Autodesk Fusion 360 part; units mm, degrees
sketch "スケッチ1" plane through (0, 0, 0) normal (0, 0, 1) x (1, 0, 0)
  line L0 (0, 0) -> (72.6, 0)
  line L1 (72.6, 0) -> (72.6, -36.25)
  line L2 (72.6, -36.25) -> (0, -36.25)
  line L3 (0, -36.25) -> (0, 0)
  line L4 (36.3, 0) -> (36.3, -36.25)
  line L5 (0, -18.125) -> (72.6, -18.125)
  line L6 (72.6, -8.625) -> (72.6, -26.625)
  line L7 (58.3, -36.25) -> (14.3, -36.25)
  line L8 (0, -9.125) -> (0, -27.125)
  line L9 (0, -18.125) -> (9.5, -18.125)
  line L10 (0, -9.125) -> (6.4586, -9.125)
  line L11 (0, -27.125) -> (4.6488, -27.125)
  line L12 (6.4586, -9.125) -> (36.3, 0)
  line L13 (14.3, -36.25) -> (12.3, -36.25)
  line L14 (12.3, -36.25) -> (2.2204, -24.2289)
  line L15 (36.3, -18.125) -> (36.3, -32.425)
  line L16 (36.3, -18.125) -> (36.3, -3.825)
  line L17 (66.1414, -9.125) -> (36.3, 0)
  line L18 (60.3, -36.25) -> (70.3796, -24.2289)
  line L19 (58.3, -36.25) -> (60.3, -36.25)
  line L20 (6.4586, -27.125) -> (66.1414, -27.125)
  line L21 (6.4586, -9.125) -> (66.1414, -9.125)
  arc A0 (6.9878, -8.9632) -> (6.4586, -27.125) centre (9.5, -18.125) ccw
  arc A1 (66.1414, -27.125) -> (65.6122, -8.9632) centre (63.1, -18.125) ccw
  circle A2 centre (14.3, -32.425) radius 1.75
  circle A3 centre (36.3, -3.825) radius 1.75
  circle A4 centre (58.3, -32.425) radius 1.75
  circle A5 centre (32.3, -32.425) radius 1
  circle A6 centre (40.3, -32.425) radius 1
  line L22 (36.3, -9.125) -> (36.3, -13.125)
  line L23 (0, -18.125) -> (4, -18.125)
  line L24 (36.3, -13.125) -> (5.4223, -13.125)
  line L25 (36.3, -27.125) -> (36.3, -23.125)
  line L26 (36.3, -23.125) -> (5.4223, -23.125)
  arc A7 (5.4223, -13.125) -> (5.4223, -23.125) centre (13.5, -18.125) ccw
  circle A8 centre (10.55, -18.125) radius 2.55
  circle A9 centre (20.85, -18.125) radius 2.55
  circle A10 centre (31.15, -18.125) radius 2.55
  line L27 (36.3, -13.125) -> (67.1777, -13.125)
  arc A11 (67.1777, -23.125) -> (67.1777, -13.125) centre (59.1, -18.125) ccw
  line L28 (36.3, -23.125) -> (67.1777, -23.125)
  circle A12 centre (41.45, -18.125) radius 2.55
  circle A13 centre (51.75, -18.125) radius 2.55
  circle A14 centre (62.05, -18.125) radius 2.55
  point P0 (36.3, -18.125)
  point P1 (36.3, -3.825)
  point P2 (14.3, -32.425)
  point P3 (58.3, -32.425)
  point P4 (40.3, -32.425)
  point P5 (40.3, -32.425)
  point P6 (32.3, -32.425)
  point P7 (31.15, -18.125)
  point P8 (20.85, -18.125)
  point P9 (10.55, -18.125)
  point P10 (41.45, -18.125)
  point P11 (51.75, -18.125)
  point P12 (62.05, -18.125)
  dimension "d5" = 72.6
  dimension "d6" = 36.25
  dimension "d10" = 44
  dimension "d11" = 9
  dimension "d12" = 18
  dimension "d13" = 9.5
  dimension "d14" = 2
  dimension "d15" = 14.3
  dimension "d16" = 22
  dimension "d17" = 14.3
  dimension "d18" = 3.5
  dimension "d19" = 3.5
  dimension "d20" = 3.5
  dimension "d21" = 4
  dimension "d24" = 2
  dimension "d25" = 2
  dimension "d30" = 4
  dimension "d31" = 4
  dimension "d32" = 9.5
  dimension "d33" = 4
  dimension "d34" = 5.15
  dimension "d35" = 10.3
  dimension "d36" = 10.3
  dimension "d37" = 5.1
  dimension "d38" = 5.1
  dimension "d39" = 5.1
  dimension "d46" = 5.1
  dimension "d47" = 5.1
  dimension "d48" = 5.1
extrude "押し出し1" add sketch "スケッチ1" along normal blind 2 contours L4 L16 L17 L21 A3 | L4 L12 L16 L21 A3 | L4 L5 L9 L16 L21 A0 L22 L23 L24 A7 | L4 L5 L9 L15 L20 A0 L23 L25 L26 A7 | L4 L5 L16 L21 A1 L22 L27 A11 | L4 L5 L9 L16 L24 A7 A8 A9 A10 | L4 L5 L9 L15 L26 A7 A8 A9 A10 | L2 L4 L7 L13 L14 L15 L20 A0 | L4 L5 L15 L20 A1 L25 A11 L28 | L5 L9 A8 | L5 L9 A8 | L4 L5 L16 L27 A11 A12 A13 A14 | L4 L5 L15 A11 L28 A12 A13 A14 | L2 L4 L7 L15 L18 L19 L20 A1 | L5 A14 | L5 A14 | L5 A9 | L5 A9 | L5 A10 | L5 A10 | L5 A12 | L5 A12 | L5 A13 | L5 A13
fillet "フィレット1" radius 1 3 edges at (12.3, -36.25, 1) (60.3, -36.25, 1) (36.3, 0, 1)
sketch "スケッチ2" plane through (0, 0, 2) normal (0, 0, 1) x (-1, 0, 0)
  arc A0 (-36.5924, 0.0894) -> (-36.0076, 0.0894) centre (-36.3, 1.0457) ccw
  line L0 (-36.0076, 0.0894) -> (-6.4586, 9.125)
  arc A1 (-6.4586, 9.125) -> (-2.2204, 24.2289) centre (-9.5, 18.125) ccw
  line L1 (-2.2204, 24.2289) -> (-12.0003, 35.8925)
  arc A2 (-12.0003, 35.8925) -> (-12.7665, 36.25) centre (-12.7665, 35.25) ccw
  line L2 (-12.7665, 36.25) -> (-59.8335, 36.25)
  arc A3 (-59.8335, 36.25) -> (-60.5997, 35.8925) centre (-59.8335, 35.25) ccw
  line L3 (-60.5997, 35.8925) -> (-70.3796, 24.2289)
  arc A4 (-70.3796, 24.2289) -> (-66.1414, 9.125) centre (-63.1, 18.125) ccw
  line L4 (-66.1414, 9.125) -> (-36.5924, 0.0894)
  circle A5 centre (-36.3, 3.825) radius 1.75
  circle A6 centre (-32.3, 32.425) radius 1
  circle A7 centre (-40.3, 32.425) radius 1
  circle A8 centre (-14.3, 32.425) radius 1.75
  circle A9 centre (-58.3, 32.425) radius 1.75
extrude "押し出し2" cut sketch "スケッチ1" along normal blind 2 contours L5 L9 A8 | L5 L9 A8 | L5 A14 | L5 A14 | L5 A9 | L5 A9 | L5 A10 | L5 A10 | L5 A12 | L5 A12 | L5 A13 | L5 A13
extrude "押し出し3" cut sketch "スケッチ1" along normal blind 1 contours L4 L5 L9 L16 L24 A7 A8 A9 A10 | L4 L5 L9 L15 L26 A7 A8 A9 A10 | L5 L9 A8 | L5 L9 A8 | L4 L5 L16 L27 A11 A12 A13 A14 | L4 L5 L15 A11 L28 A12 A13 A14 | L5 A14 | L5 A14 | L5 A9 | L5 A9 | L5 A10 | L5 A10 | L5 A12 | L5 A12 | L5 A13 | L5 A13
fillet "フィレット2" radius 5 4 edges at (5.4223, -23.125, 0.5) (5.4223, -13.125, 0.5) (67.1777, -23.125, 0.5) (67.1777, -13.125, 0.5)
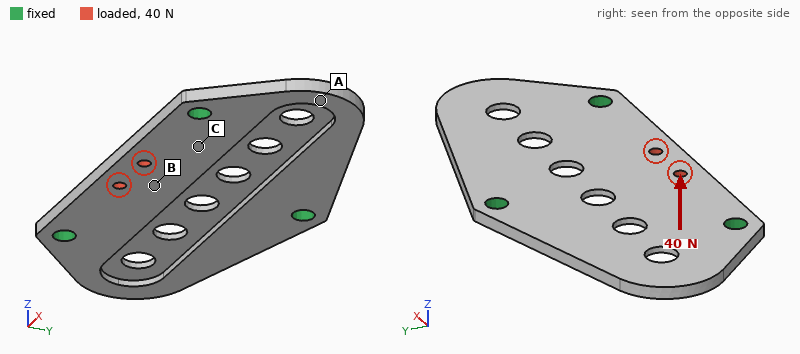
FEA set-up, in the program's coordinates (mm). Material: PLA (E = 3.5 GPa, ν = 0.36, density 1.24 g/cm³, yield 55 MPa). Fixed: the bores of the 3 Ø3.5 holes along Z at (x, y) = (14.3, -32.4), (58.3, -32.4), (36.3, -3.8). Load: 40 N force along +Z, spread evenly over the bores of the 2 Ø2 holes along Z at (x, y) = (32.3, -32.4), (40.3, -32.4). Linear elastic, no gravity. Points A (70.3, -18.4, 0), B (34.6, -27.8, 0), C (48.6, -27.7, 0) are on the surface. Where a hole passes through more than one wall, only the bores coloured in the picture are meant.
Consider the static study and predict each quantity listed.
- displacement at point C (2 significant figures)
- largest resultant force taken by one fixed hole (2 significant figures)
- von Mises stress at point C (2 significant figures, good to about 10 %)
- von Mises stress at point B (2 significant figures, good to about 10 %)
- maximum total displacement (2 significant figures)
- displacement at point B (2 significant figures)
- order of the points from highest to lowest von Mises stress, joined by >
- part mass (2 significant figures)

0.15 mm
19 N
7.7 MPa
12 MPa
0.58 mm
0.36 mm
B > C > A
4.0 g
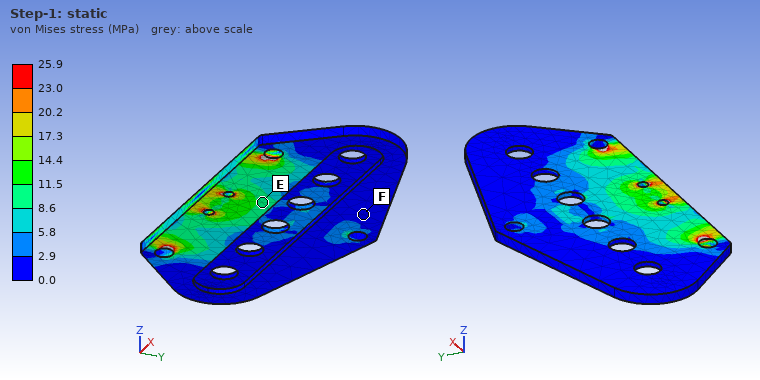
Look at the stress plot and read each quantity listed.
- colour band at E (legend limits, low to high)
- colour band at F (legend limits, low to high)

8.6 to 11.5 MPa
0.0 to 2.9 MPa
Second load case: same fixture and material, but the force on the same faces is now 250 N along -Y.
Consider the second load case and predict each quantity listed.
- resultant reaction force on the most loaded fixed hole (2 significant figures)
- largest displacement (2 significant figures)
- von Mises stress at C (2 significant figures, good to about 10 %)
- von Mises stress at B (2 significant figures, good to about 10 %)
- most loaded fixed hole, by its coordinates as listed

100 N
0.10 mm
7.0 MPa
5.0 MPa
(36.3, -3.8)
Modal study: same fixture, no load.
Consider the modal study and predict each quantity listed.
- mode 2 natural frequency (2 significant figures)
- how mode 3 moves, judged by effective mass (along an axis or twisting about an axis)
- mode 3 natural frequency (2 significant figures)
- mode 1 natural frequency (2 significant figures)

1200 Hz
along Z
2000 Hz
1200 Hz
